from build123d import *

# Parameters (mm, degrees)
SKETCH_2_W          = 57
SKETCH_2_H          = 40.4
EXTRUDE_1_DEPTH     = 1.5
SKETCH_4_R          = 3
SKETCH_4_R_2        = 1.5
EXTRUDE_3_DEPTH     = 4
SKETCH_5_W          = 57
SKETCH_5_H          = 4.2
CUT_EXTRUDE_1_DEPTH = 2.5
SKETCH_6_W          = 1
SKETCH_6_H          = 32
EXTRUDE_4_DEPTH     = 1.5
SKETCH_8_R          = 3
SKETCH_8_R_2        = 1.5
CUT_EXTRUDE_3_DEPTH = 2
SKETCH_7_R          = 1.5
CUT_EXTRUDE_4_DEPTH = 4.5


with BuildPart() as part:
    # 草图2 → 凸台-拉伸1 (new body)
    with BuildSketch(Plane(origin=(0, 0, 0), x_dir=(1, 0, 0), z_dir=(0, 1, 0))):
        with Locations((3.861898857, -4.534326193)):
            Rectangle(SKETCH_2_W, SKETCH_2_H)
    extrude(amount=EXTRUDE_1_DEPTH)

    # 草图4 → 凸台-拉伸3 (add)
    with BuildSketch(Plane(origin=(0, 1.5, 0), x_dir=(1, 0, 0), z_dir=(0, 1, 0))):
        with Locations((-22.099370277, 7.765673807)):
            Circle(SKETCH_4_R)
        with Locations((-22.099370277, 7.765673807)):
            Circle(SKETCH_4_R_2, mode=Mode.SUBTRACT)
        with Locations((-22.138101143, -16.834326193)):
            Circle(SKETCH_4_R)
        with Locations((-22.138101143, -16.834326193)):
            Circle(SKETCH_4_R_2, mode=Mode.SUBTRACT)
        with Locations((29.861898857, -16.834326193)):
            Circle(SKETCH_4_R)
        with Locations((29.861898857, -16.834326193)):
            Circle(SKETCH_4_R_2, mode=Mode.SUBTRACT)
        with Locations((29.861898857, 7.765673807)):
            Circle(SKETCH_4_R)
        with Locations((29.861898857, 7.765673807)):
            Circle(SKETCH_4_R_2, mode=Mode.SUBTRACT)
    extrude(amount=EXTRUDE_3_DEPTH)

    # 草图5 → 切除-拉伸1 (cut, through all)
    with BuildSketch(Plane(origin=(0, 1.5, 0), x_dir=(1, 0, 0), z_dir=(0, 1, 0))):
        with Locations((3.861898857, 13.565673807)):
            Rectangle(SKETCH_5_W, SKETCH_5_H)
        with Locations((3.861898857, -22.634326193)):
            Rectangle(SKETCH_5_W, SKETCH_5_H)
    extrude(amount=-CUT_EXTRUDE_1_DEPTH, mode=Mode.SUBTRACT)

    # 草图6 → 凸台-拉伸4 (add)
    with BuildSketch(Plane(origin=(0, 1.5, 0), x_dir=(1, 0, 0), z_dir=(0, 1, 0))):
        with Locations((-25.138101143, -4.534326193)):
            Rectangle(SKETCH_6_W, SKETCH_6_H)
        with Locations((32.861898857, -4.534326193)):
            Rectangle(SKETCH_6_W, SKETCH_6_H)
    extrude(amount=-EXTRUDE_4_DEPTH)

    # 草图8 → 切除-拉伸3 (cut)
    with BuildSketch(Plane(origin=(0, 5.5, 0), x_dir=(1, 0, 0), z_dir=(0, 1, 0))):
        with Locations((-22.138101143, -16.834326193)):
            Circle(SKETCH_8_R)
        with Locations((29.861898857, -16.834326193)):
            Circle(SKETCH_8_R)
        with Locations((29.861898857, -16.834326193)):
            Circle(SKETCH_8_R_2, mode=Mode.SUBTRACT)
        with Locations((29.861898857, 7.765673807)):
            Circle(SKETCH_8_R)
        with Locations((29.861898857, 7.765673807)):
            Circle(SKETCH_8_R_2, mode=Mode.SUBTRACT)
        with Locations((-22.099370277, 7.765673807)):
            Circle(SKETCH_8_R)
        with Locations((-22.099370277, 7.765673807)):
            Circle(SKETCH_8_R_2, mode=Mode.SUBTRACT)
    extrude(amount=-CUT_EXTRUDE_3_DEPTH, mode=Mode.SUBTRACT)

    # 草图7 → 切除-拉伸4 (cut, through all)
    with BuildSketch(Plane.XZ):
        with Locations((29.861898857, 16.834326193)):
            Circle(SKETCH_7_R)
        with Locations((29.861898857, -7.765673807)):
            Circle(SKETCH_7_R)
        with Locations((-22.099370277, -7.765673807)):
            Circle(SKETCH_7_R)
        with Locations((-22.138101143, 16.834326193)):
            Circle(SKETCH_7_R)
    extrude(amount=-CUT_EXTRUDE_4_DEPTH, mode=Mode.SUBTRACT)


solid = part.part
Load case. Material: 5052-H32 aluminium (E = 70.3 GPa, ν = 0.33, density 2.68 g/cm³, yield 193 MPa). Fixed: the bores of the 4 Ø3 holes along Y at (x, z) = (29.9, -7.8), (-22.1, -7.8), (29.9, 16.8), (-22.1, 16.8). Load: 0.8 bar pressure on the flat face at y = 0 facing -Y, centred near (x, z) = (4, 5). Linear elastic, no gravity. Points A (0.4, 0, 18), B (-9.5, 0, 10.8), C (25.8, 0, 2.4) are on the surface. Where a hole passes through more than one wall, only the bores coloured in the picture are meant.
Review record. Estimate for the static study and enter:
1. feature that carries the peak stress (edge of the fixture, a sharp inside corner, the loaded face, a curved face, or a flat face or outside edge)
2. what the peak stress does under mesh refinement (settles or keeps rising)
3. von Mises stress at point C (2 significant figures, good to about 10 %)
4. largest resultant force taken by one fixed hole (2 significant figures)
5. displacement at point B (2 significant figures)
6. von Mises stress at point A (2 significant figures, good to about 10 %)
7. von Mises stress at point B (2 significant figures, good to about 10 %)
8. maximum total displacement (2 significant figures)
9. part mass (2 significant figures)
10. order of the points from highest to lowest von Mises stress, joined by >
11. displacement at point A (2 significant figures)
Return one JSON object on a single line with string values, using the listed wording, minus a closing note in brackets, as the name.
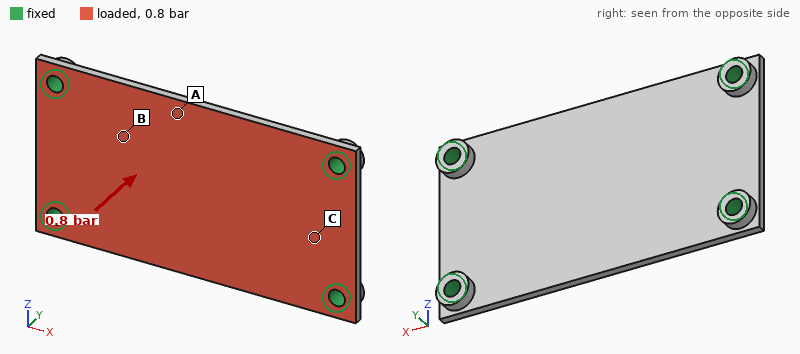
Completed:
{"feature that carries the peak stress": "edge of the fixture", "what the peak stress does under mesh refinement": "keeps rising", "von Mises stress at point C": "15 MPa", "largest resultant force taken by one fixed hole": "39 N", "displacement at point B": "38 µm", "von Mises stress at point A": "23 MPa", "von Mises stress at point B": "6.4 MPa", "maximum total displacement": "70 µm", "part mass": "7.9 g", "order of the points from highest to lowest von Mises stress, joined by >": "A > C > B", "displacement at point A": "66 µm"}
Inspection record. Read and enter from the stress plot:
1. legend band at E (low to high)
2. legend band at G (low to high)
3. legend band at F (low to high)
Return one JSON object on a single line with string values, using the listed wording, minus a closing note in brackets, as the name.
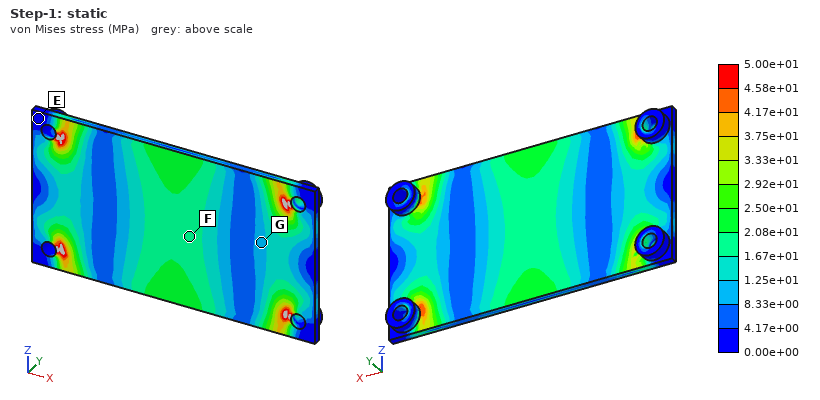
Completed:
{"legend band at E": "0.00e+00 to 4.17e+00 MPa", "legend band at G": "8.33e+00 to 1.25e+01 MPa", "legend band at F": "1.67e+01 to 2.08e+01 MPa"}
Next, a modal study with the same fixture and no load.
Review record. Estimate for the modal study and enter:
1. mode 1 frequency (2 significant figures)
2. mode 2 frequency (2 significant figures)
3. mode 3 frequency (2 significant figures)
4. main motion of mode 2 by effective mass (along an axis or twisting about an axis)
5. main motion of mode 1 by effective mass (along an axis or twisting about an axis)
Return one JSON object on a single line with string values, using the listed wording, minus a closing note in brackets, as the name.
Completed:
{"mode 1 frequency": "3100 Hz", "mode 2 frequency": "4700 Hz", "mode 3 frequency": "8300 Hz", "main motion of mode 2 by effective mass": "twisting about X", "main motion of mode 1 by effective mass": "along Y"}
